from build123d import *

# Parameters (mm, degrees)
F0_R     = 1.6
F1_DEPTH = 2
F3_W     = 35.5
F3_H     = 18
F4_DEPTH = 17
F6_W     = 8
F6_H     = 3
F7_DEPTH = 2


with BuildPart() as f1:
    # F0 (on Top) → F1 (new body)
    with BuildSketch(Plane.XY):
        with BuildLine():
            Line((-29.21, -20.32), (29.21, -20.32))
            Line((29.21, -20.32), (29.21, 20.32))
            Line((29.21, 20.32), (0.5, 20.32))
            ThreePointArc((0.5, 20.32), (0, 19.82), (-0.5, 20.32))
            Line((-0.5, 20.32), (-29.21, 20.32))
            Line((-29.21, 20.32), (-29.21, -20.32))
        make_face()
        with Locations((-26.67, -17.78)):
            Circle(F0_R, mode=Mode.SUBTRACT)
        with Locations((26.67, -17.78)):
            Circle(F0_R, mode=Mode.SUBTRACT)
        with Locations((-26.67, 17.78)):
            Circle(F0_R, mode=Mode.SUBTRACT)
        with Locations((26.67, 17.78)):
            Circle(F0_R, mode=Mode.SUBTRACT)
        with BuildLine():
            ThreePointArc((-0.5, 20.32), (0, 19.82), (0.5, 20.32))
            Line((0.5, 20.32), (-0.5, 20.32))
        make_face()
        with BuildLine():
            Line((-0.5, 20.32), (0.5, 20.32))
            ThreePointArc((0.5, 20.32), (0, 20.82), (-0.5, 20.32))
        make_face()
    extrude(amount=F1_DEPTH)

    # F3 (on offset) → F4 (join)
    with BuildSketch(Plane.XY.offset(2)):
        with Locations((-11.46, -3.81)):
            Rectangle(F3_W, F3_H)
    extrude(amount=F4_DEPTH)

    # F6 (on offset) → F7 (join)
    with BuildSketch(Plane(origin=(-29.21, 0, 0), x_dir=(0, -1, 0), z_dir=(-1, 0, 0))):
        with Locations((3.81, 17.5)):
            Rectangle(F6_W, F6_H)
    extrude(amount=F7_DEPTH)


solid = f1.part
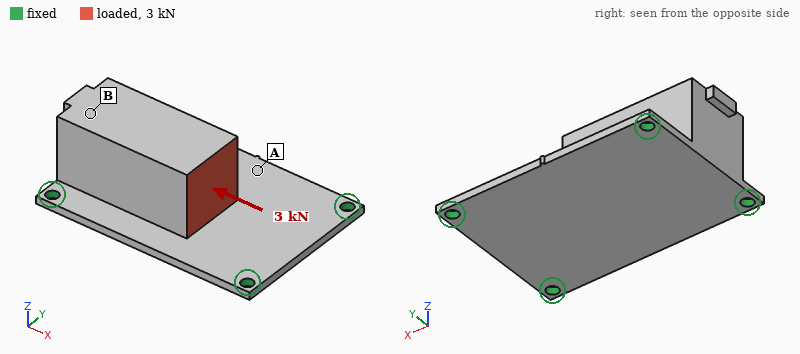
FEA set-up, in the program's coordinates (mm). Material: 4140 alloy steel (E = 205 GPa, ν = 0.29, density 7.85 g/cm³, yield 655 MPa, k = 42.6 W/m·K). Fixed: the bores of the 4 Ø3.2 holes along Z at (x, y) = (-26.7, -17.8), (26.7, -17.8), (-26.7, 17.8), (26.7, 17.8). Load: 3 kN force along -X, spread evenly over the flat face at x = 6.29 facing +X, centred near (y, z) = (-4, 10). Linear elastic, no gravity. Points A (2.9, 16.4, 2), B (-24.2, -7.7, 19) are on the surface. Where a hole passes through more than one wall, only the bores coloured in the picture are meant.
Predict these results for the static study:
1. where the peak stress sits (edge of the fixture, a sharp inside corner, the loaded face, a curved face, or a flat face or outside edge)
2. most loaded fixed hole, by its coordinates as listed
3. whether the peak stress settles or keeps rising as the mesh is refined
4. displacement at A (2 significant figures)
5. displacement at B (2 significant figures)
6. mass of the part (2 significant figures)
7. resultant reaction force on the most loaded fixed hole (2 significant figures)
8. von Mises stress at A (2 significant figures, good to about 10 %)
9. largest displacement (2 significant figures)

edge of the fixture
(-26.7, -17.8)
keeps rising
0.063 mm
0.076 mm
120 g
1.1 kN
99 MPa
0.14 mm
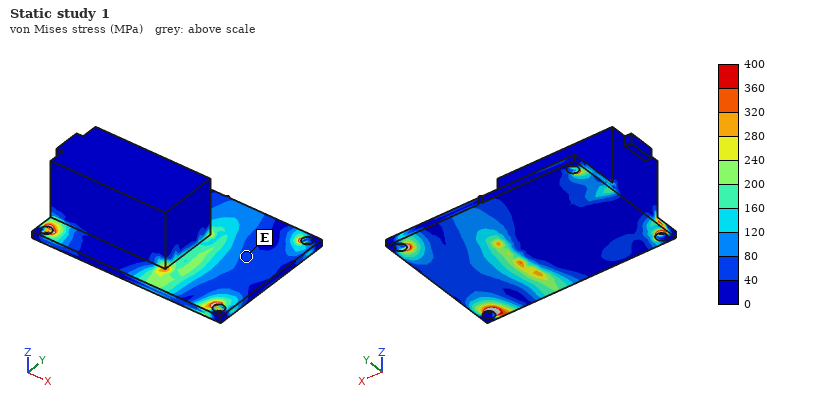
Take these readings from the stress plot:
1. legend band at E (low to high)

40 to 80 MPa
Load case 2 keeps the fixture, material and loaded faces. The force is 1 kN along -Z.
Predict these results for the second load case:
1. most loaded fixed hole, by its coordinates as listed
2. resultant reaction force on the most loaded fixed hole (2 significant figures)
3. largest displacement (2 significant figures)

(26.7, -17.8)
390 N
0.15 mm
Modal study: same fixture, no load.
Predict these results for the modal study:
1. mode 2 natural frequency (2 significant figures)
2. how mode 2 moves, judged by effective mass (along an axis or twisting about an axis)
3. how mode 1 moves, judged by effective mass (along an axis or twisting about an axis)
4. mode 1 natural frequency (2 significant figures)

3100 Hz
along Y
along Z
2000 Hz
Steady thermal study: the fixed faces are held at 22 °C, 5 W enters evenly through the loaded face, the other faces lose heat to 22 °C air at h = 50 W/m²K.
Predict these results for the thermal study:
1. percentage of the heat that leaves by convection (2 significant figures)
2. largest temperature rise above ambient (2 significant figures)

48 %
14 K
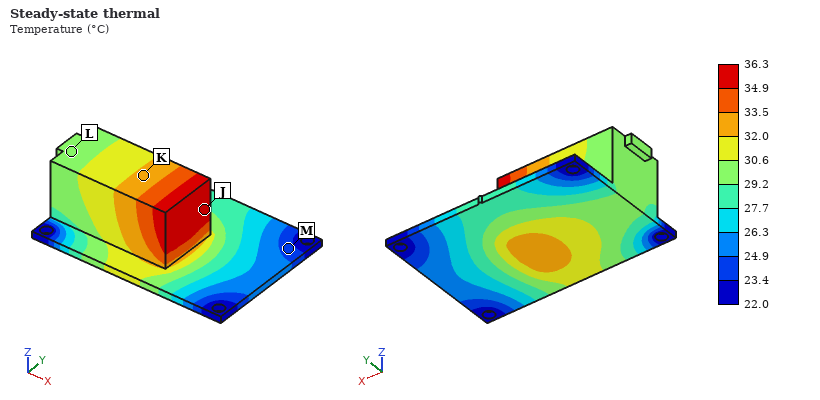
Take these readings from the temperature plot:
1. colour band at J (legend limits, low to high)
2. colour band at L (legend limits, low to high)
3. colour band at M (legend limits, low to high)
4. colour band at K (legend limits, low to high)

34.9 to 36.3 °C
29.2 to 30.6 °C
23.4 to 24.9 °C
32.0 to 33.5 °C
